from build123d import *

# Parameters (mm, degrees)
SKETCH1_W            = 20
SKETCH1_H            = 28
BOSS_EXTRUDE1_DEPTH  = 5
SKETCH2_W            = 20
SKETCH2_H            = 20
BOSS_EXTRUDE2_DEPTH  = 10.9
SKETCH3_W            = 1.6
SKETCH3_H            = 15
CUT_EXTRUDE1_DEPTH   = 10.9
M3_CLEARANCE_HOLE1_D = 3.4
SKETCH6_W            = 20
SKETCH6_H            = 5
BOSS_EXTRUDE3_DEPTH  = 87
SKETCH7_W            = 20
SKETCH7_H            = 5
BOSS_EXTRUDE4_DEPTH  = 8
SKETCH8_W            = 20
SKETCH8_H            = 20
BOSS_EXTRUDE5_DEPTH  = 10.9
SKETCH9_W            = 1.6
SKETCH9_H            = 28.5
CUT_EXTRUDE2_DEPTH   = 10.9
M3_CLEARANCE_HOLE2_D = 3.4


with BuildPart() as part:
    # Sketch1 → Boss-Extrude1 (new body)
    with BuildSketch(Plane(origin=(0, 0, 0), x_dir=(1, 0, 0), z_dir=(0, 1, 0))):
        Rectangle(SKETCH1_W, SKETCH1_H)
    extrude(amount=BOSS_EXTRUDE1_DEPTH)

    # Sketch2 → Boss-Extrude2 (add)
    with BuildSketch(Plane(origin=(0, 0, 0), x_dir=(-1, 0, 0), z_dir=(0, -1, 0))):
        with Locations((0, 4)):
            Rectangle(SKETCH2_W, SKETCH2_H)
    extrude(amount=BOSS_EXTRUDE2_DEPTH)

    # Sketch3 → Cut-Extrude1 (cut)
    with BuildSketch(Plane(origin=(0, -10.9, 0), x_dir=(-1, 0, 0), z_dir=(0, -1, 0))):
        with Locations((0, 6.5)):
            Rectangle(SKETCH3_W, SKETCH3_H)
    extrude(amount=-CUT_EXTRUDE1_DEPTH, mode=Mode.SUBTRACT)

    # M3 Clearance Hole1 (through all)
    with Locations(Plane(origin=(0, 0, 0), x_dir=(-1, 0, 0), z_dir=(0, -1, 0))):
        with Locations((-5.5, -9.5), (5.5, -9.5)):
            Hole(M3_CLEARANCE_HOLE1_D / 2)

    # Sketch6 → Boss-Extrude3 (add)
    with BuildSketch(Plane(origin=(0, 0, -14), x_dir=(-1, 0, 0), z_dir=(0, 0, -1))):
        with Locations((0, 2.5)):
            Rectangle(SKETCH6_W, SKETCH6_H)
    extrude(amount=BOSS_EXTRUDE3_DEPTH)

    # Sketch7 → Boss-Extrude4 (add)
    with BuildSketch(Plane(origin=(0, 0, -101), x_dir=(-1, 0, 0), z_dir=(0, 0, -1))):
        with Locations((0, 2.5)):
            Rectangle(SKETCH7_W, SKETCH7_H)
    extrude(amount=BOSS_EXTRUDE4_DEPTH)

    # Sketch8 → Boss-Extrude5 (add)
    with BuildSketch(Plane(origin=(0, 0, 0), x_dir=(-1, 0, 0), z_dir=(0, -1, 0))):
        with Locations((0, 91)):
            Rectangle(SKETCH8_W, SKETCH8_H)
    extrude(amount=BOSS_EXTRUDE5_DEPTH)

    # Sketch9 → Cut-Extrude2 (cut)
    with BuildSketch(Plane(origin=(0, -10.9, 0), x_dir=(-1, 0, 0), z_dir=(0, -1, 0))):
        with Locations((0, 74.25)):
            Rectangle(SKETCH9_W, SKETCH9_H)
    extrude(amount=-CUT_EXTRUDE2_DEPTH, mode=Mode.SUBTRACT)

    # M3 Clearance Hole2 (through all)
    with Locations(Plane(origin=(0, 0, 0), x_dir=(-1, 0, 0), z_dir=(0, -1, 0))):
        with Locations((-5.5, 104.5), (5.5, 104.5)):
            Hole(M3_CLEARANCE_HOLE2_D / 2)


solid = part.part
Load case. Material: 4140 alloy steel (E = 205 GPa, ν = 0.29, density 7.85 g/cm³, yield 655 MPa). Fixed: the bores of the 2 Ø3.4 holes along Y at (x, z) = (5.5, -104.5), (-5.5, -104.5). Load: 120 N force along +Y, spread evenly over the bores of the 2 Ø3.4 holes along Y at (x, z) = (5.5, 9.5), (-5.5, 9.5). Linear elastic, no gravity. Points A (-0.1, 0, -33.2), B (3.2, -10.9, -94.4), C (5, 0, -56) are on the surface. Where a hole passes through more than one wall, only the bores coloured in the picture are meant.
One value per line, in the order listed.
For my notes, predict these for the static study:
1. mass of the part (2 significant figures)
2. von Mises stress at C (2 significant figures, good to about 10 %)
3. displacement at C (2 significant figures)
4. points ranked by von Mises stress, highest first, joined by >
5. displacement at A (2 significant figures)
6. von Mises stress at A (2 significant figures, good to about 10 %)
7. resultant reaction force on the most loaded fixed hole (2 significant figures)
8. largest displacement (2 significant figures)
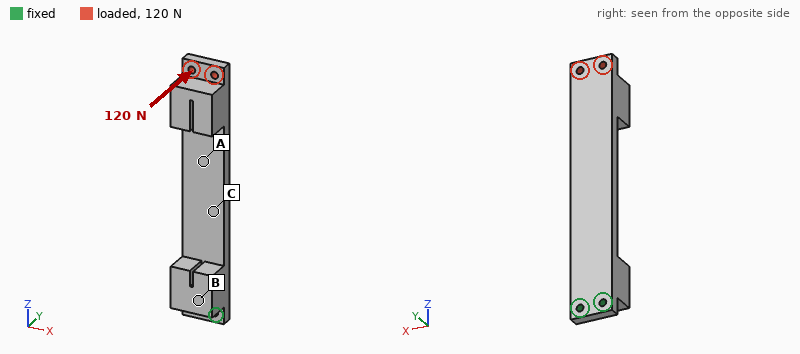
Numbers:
160 g
94 MPa
0.17 mm
C > A > B
0.40 mm
61 MPa
60 N
1.0 mm
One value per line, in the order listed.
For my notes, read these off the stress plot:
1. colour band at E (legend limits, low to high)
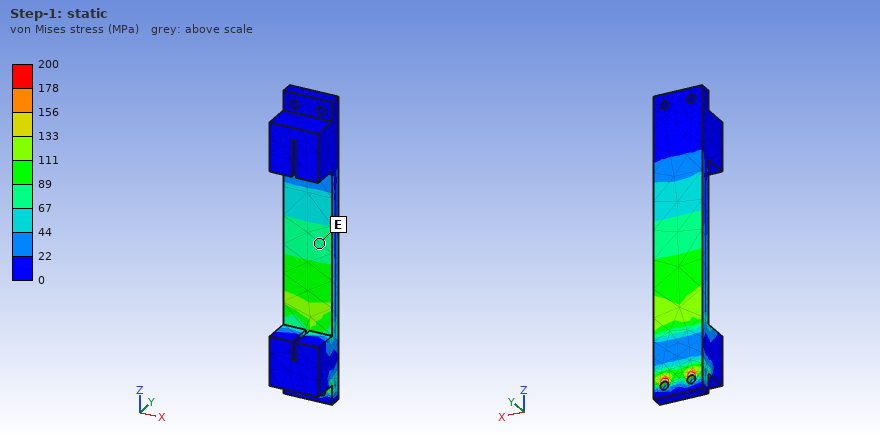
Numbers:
67 to 89 MPa
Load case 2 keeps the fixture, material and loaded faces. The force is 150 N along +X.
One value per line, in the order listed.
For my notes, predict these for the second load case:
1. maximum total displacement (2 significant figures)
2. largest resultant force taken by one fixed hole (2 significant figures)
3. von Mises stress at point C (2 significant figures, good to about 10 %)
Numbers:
0.11 mm
1.3 kN
15 MPa
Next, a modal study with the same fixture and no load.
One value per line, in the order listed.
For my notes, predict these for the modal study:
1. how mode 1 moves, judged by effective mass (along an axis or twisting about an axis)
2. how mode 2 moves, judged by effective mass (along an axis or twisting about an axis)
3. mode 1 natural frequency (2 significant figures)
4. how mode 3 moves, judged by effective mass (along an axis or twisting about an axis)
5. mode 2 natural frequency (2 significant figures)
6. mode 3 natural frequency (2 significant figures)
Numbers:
along Y
along X
270 Hz
along Y
880 Hz
1800 Hz
